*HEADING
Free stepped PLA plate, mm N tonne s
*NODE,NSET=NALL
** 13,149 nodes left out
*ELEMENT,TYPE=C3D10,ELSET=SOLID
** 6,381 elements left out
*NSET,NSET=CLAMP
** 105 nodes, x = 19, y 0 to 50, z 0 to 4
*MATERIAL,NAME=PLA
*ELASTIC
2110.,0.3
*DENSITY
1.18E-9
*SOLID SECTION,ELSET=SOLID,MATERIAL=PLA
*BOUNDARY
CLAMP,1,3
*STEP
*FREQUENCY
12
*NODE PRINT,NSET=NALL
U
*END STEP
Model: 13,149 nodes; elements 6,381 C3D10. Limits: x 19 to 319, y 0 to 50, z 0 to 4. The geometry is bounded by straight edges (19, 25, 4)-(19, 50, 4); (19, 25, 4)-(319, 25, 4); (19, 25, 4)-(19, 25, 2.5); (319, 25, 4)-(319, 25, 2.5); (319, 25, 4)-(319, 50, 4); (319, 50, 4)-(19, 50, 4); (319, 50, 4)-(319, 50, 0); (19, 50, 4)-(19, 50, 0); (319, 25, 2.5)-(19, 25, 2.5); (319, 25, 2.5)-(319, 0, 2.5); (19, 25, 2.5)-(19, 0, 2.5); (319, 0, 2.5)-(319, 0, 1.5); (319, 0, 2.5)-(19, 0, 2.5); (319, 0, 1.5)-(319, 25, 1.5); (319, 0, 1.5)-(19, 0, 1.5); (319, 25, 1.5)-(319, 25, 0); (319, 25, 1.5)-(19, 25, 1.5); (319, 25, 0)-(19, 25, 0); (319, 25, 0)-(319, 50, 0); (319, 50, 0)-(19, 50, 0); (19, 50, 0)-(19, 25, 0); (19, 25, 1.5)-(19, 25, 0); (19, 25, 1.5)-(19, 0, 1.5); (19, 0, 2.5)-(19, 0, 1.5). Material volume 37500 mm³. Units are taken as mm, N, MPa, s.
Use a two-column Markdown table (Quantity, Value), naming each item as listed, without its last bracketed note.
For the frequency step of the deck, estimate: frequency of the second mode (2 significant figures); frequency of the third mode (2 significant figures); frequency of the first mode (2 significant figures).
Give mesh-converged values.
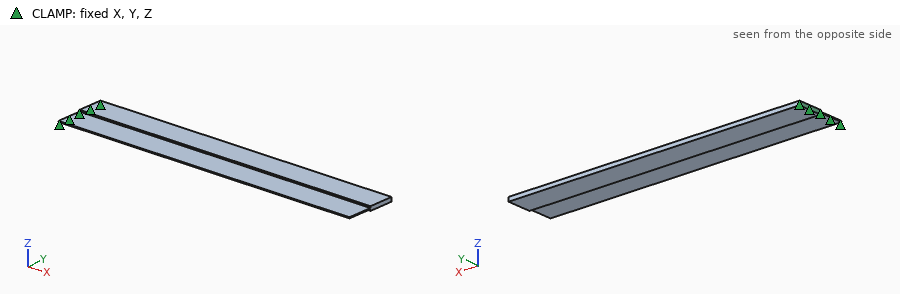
| Quantity | Value |
|---|---|
| frequency of the second mode | 54 Hz |
| frequency of the third mode | 100 Hz |
| frequency of the first mode | 8.7 Hz |
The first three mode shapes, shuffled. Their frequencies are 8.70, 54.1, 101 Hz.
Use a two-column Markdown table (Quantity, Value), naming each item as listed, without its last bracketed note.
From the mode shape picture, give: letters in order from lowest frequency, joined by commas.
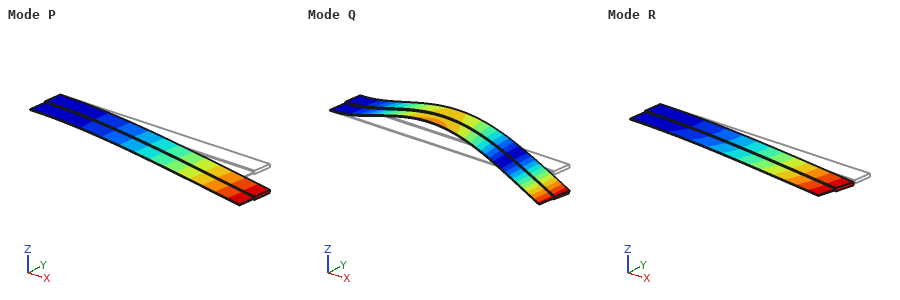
| Quantity | Value |
|---|---|
| letters in order from lowest frequency, joined by commas | P, Q, R |
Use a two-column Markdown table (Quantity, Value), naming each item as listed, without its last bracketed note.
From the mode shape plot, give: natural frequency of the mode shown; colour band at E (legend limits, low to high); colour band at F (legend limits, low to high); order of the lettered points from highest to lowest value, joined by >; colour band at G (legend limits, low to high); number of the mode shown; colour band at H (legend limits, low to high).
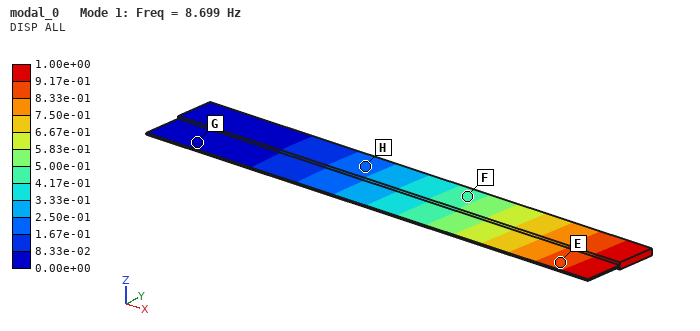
| Quantity | Value |
|---|---|
| natural frequency of the mode shown | 8.699 Hz |
| colour band at E | 8.33e-01 to 9.17e-01 |
| colour band at F | 4.17e-01 to 5.00e-01 |
| order of the lettered points from highest to lowest value, joined by > | E > F > H > G |
| colour band at G | 0.00e+00 to 8.33e-02 |
| number of the mode shown | 1 |
| colour band at H | 1.67e-01 to 2.50e-01 |
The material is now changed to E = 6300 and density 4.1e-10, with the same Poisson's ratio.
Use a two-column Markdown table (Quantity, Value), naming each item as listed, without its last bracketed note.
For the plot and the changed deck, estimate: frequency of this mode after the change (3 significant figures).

| Quantity | Value |
|---|---|
| frequency of this mode after the change | 25.5 Hz |
